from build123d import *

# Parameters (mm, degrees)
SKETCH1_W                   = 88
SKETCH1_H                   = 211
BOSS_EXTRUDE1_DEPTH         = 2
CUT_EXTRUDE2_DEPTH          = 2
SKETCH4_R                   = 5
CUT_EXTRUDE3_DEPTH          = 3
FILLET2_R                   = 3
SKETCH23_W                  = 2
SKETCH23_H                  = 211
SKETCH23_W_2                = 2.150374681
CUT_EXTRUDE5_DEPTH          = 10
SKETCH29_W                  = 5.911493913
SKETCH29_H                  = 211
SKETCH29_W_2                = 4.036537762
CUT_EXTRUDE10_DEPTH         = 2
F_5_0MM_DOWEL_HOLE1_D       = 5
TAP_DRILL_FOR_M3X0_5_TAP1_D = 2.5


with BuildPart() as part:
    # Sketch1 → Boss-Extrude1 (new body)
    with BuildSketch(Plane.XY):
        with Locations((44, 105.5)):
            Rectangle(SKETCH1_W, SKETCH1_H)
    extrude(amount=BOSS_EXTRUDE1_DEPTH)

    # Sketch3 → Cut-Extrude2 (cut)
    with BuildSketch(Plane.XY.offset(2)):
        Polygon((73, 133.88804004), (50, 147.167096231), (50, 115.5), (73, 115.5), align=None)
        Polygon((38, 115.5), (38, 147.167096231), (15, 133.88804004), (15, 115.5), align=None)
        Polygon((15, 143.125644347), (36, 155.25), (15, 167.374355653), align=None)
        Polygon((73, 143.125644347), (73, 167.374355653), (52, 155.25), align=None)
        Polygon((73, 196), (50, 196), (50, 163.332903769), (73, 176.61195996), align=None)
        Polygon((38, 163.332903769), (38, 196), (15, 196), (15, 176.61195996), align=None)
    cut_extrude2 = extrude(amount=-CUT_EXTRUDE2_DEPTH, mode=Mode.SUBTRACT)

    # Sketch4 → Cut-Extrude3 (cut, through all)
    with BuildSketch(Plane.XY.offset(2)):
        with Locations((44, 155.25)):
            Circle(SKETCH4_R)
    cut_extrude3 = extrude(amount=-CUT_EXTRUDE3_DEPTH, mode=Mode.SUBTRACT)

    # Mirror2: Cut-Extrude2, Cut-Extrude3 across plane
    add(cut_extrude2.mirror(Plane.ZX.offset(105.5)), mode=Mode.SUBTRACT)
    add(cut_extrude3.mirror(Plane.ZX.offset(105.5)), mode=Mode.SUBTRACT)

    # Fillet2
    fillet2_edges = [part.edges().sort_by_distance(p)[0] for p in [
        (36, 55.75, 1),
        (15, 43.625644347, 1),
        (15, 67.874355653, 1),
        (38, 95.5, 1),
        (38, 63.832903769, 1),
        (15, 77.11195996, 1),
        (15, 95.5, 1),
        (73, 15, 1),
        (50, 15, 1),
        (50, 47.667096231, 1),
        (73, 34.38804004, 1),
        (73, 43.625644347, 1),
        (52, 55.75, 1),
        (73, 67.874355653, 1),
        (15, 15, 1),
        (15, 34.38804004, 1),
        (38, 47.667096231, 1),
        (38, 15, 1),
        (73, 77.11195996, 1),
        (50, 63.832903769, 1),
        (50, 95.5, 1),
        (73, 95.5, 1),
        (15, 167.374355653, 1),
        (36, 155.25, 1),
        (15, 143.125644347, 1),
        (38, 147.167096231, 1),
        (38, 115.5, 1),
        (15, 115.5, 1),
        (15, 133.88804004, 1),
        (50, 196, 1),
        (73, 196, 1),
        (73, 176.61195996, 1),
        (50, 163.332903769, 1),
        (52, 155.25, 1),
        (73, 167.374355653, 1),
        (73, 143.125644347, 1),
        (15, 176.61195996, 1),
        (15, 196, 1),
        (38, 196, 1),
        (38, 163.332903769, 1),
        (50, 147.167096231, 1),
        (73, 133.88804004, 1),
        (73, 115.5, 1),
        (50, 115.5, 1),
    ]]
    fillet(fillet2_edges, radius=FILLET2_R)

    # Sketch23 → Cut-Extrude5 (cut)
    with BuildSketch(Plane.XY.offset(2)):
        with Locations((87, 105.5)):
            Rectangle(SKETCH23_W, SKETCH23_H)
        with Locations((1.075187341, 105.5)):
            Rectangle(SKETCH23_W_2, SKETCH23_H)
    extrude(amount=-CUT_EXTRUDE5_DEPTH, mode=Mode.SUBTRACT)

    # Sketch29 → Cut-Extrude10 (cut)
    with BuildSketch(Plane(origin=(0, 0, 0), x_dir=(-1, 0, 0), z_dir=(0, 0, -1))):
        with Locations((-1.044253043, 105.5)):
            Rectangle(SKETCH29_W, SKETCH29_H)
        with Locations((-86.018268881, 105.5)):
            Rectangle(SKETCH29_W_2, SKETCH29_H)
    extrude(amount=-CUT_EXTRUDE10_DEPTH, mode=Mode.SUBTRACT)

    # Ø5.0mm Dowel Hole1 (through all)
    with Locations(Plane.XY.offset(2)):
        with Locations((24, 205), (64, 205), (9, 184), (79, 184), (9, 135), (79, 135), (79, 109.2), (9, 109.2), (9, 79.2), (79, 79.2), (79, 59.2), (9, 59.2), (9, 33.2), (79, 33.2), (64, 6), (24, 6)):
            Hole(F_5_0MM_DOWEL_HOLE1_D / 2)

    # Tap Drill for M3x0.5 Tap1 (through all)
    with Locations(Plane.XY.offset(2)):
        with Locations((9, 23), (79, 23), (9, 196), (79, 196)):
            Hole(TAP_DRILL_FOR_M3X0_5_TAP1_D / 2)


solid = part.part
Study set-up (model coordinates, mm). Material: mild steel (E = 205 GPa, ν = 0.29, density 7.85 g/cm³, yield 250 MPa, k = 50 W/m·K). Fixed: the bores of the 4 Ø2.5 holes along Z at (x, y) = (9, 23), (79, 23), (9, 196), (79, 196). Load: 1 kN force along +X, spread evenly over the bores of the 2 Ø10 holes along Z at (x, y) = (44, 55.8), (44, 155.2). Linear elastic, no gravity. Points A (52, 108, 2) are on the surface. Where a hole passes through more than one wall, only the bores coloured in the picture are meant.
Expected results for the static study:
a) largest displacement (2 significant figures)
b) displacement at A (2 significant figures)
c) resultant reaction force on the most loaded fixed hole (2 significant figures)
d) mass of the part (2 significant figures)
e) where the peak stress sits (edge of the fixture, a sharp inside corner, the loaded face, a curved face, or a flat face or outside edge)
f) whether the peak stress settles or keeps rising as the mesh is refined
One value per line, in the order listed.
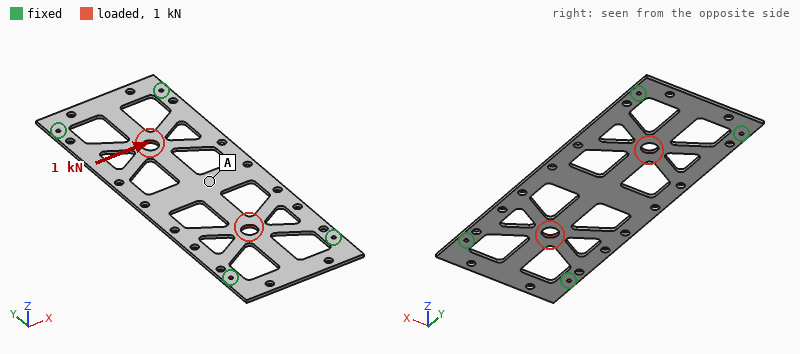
15 µm
13 µm
350 N
170 g
edge of the fixture
keeps rising
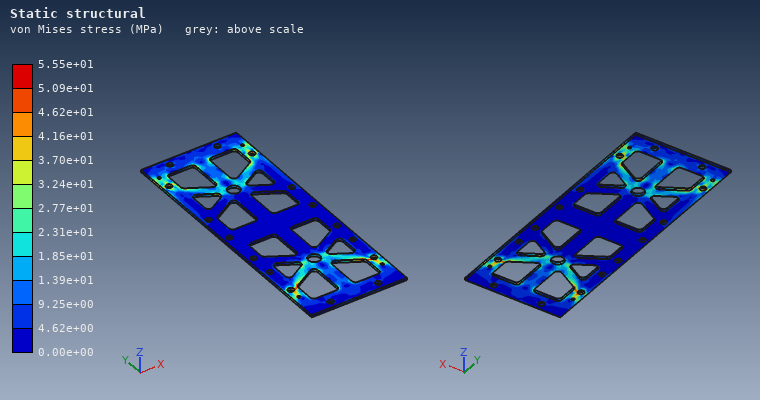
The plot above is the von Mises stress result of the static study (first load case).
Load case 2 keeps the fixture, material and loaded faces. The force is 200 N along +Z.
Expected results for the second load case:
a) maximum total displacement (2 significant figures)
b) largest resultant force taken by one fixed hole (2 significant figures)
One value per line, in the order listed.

0.61 mm
52 N
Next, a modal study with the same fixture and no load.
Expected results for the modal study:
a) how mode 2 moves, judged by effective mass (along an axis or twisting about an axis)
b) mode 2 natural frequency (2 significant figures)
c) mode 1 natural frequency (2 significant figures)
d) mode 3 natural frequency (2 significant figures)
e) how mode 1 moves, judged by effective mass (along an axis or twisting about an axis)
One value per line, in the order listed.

twisting about Y
500 Hz
270 Hz
740 Hz
along Z
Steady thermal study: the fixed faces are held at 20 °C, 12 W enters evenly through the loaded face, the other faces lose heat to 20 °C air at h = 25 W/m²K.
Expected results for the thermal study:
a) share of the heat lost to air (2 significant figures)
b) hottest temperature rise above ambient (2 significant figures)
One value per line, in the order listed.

75 %
41 K
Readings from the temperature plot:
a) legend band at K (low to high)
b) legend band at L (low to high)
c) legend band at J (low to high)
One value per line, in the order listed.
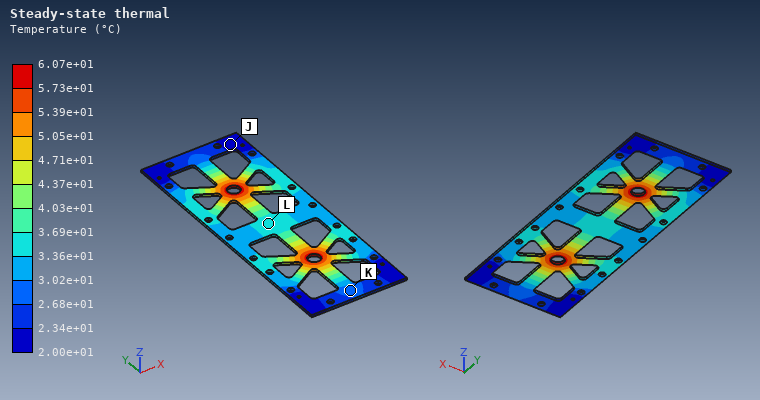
2.68e+01 to 3.02e+01 °C
3.36e+01 to 3.69e+01 °C
2.00e+01 to 2.34e+01 °C
